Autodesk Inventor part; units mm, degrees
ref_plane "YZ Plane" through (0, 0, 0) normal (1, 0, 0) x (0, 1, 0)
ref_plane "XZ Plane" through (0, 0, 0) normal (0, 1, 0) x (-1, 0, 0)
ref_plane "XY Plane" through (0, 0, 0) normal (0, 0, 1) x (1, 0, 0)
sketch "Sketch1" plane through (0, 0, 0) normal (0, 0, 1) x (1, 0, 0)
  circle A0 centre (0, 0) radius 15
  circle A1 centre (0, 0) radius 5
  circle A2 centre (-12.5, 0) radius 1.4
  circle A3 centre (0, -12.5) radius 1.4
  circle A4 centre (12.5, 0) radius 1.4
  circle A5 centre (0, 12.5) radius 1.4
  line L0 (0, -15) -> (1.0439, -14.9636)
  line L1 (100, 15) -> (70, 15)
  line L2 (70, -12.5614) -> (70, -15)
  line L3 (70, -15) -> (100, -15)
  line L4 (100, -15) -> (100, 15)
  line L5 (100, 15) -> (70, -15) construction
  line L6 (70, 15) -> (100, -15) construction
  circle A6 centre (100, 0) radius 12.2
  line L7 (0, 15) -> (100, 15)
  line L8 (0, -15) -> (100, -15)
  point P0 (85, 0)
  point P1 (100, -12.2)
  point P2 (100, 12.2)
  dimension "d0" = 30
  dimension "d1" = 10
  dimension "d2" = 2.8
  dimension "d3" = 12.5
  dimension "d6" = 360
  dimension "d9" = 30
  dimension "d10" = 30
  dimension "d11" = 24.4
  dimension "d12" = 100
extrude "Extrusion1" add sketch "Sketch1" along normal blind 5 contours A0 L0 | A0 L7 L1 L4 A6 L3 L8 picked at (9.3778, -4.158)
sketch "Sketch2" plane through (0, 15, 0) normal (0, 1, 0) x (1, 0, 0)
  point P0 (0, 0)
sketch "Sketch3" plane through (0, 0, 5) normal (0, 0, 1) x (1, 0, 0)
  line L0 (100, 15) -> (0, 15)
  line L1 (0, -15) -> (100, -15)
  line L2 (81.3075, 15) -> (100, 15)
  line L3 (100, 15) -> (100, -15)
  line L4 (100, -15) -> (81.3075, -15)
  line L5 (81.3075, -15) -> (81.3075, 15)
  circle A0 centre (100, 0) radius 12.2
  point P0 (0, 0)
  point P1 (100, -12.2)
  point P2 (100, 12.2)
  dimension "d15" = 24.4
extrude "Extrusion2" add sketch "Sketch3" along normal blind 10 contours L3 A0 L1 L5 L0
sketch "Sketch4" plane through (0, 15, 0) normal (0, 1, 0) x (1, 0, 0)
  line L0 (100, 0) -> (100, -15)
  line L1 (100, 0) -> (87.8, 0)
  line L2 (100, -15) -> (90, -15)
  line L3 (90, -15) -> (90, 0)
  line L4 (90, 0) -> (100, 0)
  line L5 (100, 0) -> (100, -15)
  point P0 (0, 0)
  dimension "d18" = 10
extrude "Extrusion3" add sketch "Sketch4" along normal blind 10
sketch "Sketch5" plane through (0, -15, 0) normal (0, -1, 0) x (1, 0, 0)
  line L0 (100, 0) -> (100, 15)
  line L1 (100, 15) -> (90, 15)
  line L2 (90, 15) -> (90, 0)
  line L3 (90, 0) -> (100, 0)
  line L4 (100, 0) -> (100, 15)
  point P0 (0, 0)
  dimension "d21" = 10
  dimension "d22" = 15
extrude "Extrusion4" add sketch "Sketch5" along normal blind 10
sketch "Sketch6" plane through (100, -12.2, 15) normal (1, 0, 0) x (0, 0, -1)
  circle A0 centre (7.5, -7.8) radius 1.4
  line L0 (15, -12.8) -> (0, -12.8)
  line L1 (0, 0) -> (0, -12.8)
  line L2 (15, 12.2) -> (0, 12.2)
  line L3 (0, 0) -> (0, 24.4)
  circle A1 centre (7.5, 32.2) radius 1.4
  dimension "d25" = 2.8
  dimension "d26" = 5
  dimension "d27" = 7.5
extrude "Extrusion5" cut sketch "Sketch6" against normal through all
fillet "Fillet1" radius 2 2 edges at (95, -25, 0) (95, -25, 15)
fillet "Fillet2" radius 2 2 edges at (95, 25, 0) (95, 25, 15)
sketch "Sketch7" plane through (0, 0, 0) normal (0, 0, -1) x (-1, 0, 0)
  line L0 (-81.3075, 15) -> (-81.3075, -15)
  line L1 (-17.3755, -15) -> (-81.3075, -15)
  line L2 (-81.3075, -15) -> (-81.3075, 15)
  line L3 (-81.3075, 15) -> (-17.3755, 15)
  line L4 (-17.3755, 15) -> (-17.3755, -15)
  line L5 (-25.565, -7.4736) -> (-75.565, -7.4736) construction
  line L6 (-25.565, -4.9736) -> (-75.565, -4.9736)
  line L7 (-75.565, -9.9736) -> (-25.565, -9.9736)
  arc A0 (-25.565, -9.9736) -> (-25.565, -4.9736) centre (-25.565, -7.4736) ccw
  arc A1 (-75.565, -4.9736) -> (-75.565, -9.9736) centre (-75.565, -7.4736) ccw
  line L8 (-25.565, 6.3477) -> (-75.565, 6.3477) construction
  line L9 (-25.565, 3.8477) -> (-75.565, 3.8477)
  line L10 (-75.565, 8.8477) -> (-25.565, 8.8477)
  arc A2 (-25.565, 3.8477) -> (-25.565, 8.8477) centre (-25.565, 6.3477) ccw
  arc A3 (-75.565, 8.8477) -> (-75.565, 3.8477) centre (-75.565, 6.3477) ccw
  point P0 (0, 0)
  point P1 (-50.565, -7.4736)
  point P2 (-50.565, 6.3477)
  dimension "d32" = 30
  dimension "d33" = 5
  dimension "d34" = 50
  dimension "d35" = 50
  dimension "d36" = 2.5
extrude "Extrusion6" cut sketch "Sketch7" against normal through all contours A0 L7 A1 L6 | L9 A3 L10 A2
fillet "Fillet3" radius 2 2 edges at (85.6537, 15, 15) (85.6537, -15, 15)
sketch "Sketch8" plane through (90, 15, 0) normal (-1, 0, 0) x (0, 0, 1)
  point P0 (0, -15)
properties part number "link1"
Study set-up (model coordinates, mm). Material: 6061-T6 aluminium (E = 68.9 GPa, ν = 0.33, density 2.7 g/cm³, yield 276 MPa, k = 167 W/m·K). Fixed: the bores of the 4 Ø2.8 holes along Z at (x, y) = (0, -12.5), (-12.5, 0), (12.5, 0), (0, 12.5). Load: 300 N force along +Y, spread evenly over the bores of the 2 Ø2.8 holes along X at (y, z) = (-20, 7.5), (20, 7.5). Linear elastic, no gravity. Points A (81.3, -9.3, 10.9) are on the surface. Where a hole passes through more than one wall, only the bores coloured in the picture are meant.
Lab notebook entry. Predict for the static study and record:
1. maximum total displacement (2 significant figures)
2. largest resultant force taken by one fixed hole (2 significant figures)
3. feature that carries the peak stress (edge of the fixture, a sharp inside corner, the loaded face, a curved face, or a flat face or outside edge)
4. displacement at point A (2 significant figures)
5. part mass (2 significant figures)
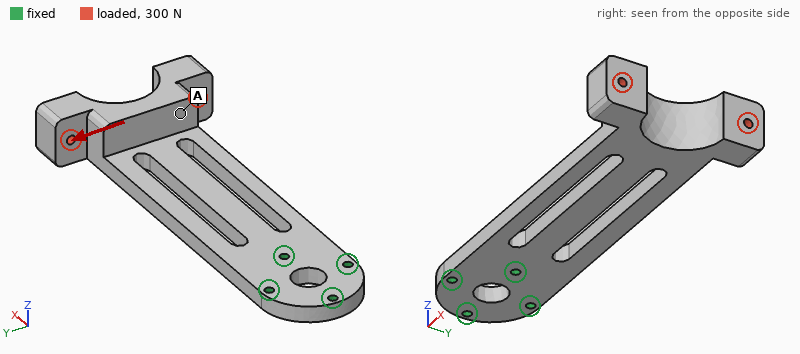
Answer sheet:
0.40 mm
840 N
a curved face
0.31 mm
50 g
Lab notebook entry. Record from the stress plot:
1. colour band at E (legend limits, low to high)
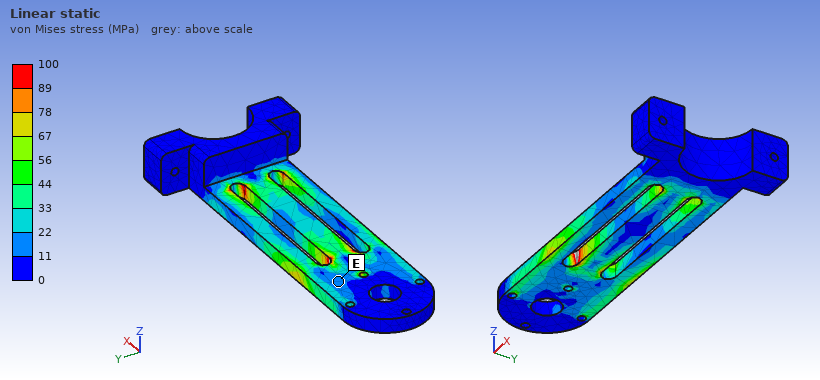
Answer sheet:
11 to 22 MPa
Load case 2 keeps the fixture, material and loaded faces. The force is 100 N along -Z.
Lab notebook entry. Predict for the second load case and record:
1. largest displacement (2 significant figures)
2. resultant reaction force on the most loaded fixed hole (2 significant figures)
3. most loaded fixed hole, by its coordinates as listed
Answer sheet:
1.3 mm
460 N
(12.5, 0)
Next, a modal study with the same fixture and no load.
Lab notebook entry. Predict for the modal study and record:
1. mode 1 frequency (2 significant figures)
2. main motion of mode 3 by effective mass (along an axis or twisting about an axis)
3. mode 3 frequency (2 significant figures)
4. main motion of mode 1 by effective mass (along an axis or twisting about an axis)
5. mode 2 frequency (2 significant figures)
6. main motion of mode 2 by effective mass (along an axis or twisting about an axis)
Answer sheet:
320 Hz
along Y
1200 Hz
along Z
900 Hz
along Y
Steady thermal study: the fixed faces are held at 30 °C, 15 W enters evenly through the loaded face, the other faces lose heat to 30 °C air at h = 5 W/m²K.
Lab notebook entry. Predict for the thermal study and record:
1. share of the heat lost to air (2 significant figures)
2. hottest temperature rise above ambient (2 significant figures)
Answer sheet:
11 %
63 K
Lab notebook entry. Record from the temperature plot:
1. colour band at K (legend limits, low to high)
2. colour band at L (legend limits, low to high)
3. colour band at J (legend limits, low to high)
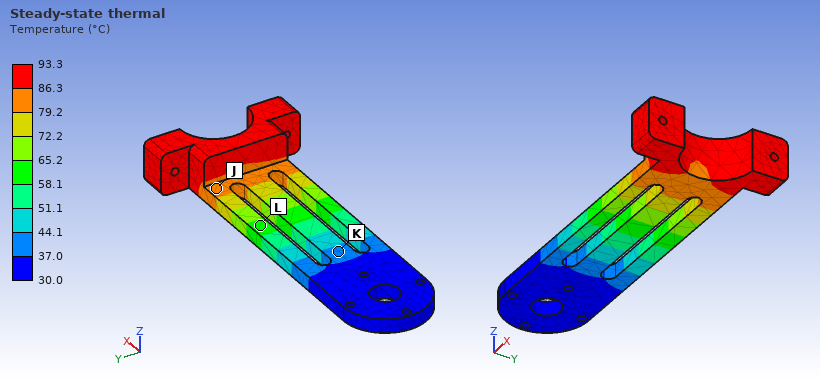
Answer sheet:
37.0 to 44.1 °C
58.1 to 65.2 °C
79.2 to 86.3 °C
